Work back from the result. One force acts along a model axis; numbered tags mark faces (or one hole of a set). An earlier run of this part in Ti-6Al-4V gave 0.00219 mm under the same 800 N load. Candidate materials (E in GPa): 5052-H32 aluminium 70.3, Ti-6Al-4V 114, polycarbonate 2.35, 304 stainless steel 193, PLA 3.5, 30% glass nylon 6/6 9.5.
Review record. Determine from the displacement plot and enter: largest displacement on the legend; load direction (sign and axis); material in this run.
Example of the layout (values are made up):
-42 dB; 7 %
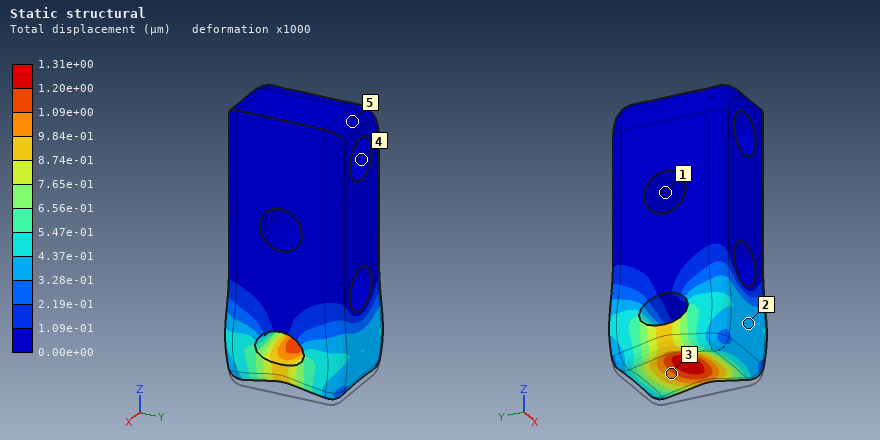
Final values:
1.31e+00 µm; +Z; 304 stainless steel
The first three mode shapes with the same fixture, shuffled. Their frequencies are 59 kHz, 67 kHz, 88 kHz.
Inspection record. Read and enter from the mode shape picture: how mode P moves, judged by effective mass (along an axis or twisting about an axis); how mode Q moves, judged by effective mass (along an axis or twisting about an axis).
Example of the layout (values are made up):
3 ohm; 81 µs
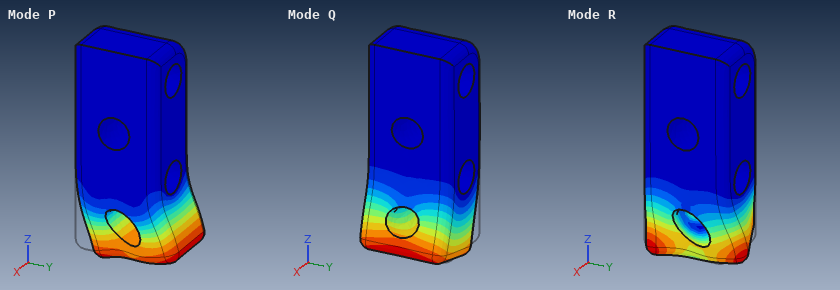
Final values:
along Y; along X
